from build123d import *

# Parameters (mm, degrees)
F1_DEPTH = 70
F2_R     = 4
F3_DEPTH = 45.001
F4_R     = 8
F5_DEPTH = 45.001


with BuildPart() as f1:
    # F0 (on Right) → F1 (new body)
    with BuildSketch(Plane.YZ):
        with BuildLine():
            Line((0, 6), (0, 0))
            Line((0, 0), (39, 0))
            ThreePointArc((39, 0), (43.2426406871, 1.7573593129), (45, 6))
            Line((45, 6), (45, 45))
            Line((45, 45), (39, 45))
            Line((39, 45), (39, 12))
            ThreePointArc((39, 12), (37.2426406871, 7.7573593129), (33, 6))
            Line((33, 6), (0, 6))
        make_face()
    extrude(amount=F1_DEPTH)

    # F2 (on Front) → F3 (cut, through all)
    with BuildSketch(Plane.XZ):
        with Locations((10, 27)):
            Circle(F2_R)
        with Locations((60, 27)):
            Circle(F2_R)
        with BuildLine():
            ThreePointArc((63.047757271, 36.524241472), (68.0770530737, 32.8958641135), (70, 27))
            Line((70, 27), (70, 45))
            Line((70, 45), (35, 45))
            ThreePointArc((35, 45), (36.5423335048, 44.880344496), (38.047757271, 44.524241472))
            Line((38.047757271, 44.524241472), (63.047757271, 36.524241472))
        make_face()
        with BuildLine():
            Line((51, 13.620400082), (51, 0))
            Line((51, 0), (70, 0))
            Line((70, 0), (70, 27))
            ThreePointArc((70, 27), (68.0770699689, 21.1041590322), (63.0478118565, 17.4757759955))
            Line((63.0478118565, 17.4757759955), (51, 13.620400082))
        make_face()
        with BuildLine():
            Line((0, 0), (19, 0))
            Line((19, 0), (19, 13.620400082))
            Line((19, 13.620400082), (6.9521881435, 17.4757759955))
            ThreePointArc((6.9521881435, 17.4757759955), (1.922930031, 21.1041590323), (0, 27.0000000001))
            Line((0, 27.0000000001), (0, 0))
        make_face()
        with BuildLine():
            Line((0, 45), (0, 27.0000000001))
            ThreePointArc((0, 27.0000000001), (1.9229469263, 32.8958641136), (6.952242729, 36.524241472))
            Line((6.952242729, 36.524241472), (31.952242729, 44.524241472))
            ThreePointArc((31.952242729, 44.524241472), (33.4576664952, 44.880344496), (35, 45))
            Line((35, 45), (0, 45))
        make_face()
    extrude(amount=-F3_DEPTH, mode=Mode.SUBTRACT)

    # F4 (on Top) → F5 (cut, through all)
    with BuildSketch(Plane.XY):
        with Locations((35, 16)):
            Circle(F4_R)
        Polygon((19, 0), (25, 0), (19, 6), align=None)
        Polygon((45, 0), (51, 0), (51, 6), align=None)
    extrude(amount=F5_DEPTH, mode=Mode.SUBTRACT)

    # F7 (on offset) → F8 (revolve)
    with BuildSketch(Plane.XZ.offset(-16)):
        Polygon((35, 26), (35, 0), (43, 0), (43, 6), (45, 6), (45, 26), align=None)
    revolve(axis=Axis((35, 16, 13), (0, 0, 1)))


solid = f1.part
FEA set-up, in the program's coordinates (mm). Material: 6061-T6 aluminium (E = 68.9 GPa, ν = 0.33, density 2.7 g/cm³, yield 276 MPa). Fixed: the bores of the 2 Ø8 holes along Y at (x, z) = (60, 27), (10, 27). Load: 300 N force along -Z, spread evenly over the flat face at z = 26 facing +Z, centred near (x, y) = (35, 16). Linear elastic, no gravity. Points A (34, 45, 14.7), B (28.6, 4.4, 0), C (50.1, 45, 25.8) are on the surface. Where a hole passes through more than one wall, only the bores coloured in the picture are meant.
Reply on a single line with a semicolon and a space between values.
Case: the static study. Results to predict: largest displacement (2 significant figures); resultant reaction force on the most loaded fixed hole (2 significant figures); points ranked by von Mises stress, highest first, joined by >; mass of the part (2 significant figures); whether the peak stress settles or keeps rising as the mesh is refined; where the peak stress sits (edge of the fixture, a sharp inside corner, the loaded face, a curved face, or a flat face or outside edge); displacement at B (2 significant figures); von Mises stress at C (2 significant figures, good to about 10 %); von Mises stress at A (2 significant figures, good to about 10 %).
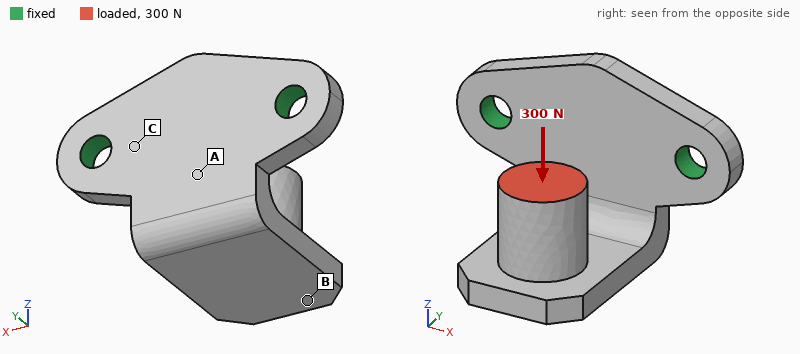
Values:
0.22 mm; 160 N; A > C > B; 69 g; keeps rising; a sharp inside corner; 0.20 mm; 17 MPa; 30 MPa
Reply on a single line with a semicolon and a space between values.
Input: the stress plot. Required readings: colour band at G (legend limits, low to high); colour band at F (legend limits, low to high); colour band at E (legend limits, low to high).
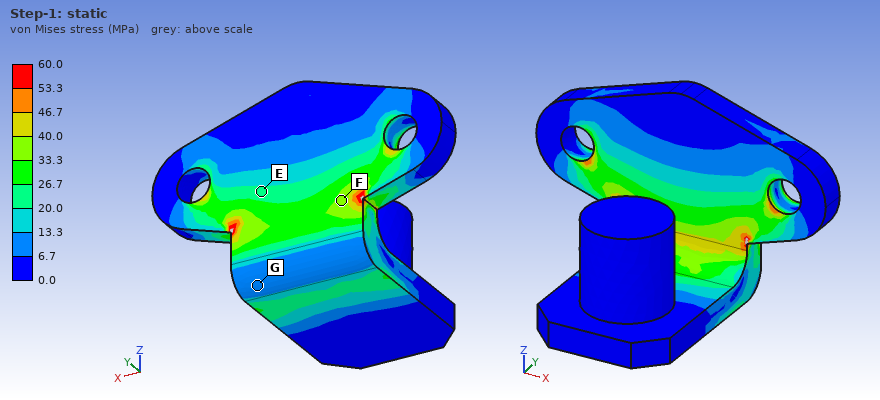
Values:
6.7 to 13.3 MPa; 33.3 to 40.0 MPa; 20.0 to 26.7 MPa
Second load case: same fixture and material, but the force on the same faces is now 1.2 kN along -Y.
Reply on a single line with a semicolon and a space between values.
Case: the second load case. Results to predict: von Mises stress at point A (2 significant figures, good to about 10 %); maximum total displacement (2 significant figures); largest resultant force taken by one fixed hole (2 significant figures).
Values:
60 MPa; 0.55 mm; 600 N
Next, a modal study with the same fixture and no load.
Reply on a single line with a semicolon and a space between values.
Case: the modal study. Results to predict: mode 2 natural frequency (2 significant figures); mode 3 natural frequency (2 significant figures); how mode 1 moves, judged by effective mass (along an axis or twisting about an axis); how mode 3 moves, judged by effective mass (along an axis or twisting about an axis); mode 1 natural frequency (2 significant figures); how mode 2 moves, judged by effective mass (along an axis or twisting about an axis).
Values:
2200 Hz; 3000 Hz; along Z; along Y; 1200 Hz; along X
